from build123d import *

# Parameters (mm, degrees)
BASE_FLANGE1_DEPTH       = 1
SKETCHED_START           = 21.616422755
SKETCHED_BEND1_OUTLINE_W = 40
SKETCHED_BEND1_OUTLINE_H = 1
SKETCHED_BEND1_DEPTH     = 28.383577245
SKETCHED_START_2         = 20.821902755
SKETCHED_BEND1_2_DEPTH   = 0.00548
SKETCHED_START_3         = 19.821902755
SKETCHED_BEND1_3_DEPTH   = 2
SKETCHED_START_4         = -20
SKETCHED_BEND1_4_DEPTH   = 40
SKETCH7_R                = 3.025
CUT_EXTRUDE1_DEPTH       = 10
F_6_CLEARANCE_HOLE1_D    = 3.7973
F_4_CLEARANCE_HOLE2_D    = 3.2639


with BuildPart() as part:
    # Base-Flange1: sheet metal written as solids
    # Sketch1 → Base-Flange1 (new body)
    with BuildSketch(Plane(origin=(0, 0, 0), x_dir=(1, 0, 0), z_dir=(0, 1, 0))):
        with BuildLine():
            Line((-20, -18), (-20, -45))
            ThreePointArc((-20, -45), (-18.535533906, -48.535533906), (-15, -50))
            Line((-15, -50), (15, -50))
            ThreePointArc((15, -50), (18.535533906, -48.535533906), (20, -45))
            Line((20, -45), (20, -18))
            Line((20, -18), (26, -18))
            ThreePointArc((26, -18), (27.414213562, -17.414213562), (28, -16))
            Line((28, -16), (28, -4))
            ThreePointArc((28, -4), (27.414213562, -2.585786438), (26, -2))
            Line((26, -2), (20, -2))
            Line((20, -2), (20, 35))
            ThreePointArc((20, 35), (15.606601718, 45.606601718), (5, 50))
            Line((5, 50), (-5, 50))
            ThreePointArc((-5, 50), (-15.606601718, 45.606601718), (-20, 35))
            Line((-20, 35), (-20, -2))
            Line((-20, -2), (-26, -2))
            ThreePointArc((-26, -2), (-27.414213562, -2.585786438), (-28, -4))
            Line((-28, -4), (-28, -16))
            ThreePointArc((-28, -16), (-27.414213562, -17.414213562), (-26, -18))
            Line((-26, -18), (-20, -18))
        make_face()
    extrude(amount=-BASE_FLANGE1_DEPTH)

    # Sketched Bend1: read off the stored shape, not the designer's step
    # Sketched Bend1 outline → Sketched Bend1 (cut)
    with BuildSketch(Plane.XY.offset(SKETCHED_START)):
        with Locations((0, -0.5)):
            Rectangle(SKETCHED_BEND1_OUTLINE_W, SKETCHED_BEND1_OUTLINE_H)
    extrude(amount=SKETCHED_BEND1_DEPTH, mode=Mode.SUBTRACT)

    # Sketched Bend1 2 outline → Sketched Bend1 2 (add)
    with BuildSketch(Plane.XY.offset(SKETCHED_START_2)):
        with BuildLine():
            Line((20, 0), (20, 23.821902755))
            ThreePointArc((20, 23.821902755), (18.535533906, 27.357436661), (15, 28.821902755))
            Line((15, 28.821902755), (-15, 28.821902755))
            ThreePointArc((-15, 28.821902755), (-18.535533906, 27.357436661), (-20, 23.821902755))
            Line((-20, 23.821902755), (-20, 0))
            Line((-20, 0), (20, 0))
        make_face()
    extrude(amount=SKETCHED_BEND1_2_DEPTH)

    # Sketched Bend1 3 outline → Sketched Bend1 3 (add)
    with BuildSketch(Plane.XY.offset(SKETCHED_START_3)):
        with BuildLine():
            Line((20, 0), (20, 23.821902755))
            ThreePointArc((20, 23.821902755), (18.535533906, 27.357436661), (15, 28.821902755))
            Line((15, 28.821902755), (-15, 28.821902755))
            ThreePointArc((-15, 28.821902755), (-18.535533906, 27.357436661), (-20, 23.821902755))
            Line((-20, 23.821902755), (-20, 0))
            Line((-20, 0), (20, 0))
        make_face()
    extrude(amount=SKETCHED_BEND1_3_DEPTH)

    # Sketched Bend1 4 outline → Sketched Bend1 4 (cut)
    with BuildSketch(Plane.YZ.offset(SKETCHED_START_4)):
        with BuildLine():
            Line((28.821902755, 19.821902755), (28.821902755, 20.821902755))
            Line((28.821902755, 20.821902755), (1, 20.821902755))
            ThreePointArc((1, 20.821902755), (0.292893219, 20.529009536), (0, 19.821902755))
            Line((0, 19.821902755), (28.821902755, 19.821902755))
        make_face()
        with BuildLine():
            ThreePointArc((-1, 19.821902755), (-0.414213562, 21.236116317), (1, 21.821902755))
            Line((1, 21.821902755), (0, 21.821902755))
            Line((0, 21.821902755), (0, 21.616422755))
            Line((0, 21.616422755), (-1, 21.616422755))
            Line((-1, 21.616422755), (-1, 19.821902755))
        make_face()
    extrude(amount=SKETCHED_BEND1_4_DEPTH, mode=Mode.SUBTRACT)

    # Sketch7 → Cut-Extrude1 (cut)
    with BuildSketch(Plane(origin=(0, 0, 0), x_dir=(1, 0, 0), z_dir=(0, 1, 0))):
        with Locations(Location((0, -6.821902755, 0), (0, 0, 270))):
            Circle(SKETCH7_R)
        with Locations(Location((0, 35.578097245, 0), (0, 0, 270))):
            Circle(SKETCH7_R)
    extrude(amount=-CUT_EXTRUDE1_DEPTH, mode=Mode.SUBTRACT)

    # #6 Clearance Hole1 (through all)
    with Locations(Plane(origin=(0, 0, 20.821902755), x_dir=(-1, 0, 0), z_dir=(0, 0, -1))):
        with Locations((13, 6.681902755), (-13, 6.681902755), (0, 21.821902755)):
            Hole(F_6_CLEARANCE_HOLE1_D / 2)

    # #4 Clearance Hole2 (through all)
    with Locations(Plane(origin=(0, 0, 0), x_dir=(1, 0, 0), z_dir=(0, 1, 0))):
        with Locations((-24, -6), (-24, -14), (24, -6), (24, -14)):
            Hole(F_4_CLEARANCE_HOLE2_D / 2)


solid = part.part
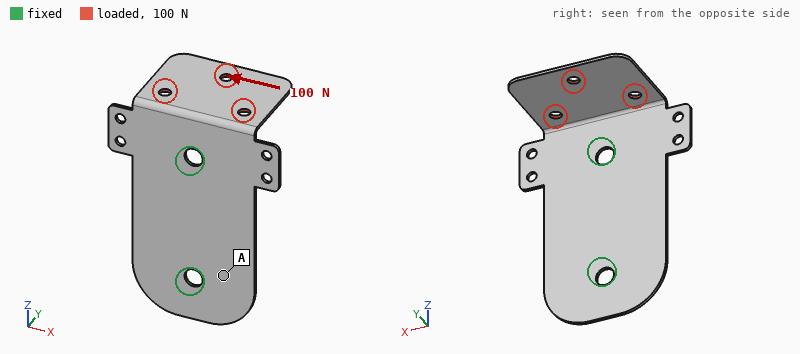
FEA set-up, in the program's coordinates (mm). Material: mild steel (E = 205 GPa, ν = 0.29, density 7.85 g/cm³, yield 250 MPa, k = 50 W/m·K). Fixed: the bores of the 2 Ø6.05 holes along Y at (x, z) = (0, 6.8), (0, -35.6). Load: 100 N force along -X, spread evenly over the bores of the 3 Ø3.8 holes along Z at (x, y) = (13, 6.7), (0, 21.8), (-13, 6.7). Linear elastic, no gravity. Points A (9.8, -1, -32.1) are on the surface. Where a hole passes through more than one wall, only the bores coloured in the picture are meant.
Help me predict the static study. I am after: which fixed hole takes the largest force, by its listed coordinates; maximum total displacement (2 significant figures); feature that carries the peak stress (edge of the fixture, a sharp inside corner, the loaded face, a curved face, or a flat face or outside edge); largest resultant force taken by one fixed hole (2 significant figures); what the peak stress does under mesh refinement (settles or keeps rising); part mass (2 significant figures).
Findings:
(0, 6.8)
0.40 mm
edge of the fixture
130 N
keeps rising
32 g
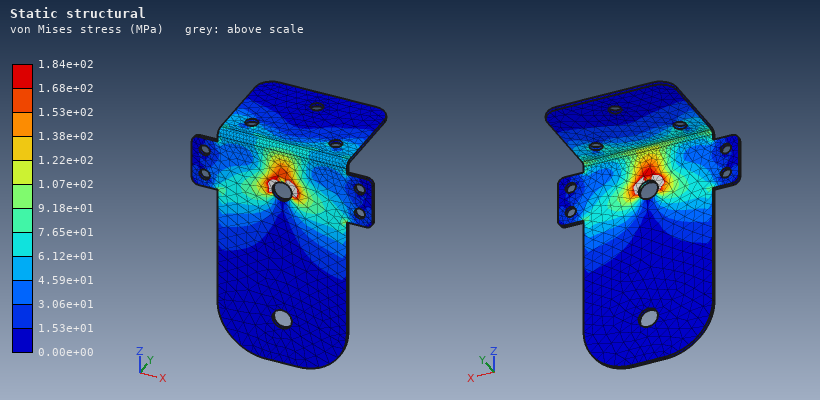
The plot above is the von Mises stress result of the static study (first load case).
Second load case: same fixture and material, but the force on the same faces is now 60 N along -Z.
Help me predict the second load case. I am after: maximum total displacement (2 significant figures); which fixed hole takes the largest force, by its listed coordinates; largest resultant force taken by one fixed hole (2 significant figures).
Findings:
0.61 mm
(0, 6.8)
48 N
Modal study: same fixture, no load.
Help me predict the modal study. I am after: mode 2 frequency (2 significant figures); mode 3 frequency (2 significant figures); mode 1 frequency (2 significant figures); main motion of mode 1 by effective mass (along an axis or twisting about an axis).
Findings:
760 Hz
1700 Hz
570 Hz
along Z
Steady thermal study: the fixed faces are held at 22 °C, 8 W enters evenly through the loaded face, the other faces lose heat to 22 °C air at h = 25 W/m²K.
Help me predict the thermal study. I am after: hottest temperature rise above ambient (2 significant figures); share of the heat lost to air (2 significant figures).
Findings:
74 K
55 %
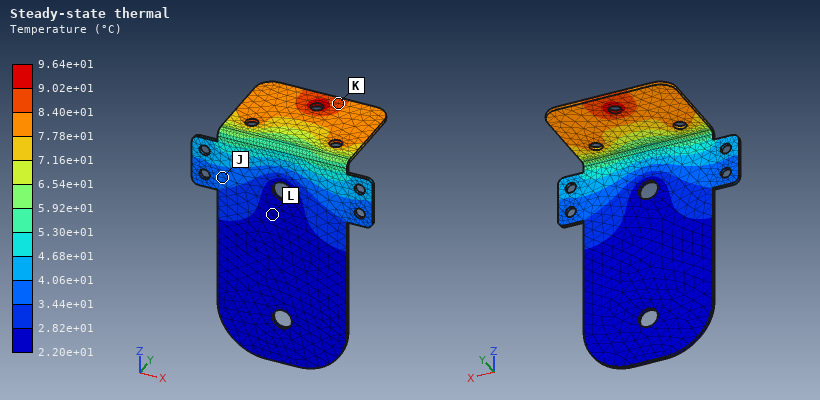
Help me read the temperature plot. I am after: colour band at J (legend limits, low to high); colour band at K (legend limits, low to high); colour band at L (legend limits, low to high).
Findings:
3.44e+01 to 4.06e+01 °C
8.40e+01 to 9.02e+01 °C
2.20e+01 to 2.82e+01 °C
